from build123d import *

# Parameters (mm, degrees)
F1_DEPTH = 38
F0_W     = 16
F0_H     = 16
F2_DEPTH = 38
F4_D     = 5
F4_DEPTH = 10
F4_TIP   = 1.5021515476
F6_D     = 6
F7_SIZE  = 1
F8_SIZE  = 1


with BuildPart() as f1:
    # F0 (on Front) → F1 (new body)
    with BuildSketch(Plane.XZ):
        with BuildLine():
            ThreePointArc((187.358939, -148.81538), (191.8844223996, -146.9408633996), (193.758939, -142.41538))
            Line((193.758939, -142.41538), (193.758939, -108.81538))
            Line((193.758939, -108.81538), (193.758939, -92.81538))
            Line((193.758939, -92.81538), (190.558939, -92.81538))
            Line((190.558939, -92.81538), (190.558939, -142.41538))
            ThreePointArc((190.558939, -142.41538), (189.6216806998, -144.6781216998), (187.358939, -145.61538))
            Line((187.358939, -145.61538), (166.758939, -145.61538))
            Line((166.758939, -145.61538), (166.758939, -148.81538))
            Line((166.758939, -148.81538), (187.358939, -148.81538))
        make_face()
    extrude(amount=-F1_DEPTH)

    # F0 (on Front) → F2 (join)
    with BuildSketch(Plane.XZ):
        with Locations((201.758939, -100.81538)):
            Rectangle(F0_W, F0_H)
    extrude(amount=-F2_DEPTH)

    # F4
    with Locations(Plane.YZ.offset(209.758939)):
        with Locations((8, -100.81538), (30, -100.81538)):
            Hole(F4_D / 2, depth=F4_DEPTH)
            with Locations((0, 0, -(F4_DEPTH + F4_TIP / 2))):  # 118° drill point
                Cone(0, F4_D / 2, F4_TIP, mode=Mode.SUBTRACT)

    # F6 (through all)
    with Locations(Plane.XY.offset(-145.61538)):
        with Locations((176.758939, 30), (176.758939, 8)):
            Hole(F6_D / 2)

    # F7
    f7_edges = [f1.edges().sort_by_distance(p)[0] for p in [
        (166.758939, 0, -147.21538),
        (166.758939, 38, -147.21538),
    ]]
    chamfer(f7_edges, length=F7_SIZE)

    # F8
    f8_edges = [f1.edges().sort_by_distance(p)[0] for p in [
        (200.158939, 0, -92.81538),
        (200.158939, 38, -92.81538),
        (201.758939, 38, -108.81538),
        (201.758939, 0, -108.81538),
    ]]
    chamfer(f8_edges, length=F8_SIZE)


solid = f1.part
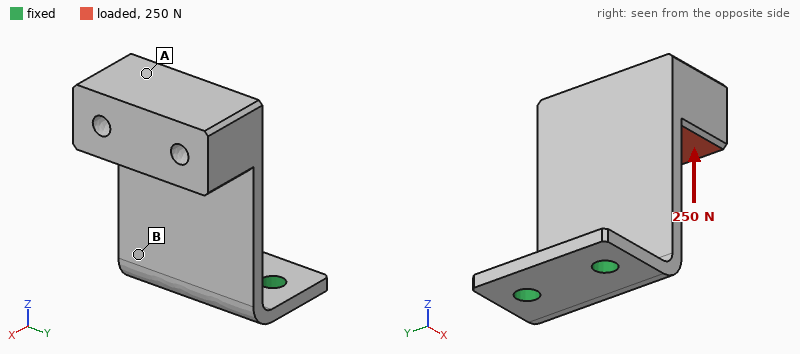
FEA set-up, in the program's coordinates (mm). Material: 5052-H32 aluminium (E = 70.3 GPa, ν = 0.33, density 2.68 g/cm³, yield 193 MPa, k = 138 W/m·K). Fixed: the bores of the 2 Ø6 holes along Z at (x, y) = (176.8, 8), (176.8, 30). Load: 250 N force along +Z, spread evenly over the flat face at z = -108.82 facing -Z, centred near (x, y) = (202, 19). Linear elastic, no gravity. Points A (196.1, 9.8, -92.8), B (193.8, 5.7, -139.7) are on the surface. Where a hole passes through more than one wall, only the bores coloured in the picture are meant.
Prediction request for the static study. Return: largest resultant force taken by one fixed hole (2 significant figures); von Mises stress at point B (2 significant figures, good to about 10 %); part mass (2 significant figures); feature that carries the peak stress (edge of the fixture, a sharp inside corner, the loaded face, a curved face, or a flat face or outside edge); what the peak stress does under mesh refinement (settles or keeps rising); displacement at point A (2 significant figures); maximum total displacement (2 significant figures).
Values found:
130 N
35 MPa
50 g
edge of the fixture
keeps rising
0.80 mm
0.88 mm
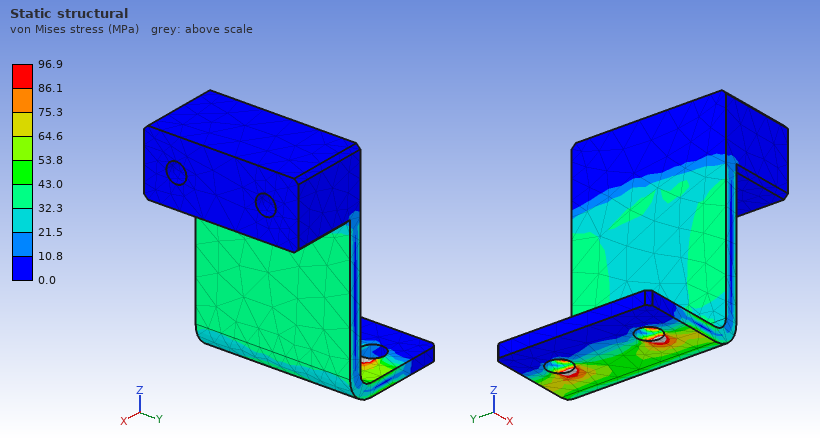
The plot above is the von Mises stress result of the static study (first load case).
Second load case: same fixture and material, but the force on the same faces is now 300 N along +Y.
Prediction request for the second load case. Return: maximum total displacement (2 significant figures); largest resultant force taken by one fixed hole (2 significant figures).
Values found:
0.27 mm
550 N
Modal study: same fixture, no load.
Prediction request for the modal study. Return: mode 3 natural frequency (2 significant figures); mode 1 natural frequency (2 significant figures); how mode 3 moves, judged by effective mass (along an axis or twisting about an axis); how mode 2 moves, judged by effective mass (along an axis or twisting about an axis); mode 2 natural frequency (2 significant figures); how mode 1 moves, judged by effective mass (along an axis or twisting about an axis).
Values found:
1400 Hz
310 Hz
twisting about Z
along Y
970 Hz
along X
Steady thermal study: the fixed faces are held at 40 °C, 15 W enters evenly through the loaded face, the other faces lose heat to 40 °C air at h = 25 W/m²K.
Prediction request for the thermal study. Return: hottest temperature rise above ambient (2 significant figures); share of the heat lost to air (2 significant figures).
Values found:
38 K
29 %
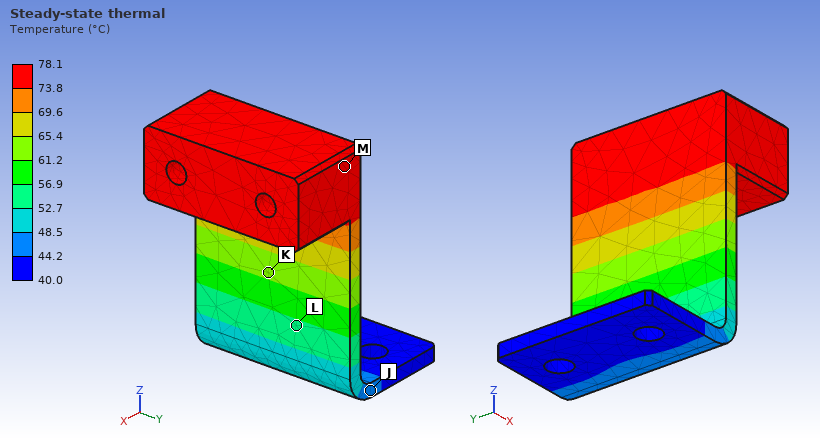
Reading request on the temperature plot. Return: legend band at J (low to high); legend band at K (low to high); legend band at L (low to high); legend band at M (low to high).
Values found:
44.2 to 48.5 °C
61.2 to 65.4 °C
52.7 to 56.9 °C
73.8 to 78.1 °C
